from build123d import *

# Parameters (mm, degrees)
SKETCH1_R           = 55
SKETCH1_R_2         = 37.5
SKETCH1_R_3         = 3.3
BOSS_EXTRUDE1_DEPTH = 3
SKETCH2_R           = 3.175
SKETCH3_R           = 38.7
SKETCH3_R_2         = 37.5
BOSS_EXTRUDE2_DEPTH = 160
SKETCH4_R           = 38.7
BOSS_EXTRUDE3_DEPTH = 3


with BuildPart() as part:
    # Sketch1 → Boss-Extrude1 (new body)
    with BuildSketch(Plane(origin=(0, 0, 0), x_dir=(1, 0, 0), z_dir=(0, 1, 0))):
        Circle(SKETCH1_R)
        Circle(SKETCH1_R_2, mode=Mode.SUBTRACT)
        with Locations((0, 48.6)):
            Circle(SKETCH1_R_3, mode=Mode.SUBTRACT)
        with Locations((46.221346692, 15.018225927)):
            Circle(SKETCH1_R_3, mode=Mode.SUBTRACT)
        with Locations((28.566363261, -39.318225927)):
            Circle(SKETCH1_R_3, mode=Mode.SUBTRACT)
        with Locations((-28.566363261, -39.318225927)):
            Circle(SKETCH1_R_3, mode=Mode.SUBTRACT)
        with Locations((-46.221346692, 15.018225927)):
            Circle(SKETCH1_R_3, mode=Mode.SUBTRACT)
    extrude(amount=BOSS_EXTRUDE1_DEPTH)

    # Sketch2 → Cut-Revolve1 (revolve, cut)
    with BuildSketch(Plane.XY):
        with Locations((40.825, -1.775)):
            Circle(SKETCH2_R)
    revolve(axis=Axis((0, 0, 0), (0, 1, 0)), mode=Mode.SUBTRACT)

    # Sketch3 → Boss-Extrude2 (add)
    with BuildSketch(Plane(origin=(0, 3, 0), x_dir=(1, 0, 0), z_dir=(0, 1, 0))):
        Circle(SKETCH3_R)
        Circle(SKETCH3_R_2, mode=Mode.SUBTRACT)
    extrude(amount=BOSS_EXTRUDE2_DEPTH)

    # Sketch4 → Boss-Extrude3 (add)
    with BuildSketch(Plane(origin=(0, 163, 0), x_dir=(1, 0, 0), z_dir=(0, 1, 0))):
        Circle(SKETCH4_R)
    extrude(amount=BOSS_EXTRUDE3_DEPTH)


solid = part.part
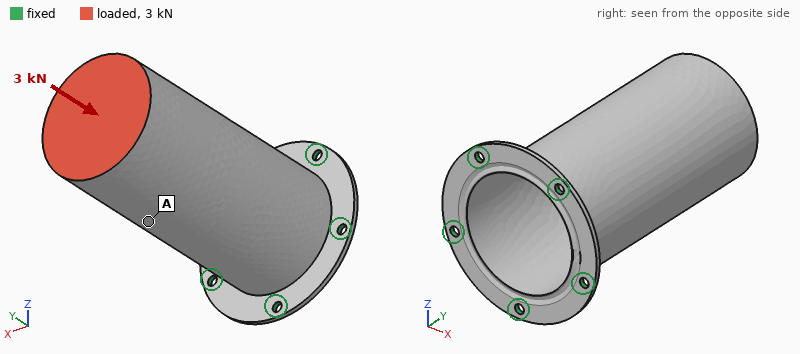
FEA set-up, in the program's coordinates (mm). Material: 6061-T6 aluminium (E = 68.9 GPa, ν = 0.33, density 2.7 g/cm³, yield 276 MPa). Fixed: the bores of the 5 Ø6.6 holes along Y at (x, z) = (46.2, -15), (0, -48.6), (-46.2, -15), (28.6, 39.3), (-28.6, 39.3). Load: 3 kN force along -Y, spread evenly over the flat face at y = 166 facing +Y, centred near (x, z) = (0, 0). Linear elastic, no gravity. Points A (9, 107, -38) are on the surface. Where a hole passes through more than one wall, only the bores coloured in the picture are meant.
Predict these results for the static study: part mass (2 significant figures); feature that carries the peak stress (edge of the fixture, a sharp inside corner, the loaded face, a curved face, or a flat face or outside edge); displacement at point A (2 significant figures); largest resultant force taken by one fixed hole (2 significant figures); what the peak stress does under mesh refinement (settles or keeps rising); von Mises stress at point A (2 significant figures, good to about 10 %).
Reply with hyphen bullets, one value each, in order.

- 200 g
- edge of the fixture
- 0.058 mm
- 650 N
- keeps rising
- 10 MPa
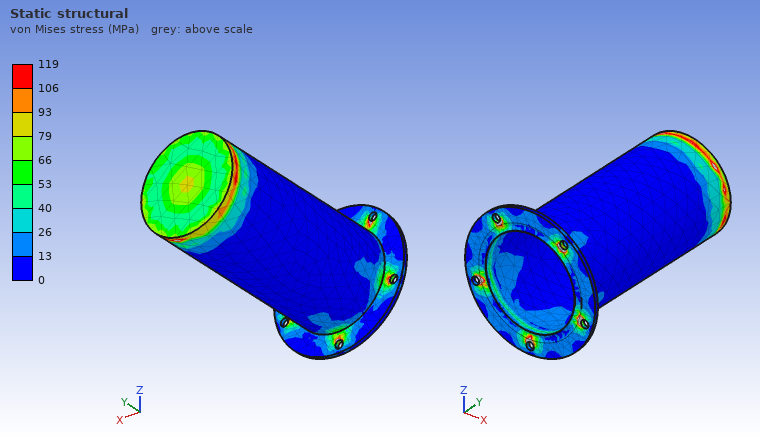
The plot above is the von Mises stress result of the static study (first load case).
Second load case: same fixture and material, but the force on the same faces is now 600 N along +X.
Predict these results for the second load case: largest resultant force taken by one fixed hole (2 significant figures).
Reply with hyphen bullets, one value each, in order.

- 940 N
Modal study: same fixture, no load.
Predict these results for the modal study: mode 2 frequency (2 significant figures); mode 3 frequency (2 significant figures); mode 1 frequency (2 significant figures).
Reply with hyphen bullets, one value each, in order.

- 740 Hz
- 2100 Hz
- 730 Hz
